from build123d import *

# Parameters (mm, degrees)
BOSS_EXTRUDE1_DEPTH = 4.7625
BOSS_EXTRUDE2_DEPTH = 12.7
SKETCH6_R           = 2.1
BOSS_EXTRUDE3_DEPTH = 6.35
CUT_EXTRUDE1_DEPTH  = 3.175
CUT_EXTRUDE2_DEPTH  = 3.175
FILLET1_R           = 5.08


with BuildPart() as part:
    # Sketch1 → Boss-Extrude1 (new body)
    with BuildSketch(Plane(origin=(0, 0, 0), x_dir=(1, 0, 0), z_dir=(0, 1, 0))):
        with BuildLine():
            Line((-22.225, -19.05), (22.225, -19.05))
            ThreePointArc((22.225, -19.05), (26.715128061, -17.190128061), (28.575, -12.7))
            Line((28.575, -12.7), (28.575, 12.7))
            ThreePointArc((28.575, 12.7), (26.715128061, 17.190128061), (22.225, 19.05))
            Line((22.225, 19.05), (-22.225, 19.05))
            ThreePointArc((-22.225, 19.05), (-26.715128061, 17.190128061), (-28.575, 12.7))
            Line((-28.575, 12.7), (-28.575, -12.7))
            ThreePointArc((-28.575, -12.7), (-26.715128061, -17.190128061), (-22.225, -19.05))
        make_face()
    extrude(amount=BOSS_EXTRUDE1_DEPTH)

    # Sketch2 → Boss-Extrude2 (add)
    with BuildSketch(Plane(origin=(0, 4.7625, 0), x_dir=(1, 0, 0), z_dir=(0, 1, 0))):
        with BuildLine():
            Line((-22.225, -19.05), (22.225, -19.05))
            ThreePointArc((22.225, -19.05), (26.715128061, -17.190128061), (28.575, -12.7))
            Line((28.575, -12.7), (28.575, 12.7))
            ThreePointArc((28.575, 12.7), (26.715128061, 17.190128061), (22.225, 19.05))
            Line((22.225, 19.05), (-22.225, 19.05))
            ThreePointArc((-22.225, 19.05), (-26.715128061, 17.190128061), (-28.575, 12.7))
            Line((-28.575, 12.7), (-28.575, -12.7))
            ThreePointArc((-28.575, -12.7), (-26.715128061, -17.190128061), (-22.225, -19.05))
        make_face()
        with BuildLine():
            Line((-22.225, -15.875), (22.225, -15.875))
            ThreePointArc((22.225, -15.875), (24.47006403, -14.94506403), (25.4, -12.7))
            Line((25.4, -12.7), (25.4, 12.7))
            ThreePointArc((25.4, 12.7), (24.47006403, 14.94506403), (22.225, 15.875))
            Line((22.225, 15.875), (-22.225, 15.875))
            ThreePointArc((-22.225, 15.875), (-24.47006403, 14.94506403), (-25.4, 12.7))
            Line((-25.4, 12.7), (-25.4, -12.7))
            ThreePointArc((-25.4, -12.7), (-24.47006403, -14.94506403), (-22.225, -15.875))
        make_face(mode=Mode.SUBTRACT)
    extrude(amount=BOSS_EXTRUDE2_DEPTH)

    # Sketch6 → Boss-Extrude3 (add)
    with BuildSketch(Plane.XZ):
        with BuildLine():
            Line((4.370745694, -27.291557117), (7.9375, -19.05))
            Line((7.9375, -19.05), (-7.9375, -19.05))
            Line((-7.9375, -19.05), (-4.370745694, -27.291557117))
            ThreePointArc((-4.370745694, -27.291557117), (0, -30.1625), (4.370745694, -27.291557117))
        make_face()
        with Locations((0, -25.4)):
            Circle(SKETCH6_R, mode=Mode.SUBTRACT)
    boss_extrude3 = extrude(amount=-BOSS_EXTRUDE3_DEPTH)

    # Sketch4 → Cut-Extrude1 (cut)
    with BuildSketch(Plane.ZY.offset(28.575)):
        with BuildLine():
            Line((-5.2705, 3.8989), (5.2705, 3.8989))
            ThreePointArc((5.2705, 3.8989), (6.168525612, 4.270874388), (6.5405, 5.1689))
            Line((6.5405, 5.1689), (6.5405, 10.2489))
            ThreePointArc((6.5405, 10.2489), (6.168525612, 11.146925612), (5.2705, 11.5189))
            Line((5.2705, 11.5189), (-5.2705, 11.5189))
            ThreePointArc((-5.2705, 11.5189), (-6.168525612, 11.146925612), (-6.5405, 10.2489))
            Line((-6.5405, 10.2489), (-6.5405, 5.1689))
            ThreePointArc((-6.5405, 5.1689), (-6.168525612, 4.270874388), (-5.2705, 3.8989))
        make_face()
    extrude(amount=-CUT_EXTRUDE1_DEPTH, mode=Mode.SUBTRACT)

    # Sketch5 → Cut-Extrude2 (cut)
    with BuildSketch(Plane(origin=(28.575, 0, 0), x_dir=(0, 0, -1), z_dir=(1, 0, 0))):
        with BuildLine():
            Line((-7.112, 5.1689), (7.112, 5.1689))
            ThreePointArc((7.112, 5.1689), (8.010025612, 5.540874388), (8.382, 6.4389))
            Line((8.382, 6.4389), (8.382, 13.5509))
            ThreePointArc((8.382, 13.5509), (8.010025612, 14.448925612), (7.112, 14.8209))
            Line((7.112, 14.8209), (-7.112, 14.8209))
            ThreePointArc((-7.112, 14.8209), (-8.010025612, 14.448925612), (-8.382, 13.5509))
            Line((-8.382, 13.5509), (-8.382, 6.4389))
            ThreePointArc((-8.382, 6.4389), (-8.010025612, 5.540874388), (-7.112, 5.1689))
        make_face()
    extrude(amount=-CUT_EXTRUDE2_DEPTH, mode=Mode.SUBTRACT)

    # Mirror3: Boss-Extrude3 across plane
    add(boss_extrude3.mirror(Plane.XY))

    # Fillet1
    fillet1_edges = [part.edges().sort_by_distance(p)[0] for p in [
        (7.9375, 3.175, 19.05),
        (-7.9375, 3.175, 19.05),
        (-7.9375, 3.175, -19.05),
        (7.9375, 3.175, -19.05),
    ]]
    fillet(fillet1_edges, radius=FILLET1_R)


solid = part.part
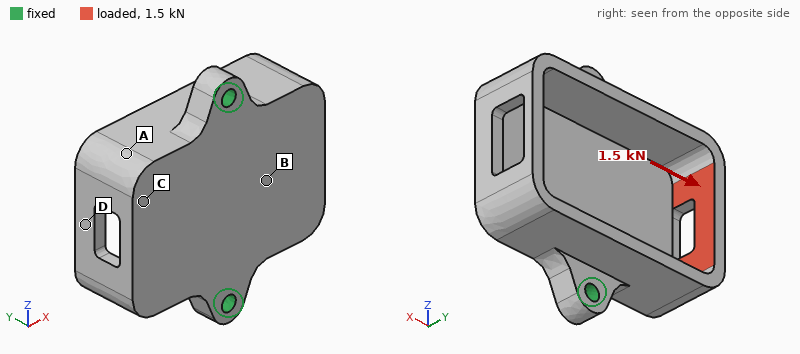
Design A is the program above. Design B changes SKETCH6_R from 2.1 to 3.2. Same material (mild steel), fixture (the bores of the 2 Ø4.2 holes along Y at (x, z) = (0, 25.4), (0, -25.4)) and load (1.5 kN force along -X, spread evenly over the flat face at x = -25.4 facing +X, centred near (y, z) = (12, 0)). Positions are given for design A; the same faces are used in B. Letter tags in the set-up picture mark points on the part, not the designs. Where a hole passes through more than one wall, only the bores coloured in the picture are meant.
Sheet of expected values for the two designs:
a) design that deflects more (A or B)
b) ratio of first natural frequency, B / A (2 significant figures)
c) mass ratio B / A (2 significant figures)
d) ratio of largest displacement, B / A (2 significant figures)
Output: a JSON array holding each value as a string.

["A", "1.2", "0.99", "0.92"]
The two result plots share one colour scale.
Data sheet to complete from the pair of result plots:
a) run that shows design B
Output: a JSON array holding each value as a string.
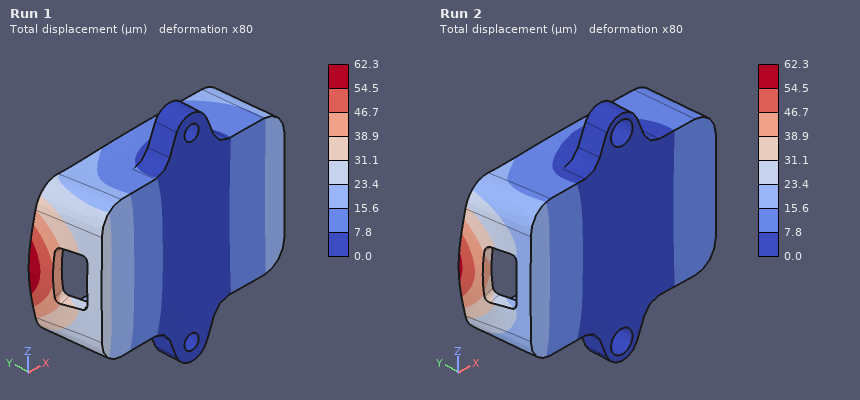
["Run 2"]
